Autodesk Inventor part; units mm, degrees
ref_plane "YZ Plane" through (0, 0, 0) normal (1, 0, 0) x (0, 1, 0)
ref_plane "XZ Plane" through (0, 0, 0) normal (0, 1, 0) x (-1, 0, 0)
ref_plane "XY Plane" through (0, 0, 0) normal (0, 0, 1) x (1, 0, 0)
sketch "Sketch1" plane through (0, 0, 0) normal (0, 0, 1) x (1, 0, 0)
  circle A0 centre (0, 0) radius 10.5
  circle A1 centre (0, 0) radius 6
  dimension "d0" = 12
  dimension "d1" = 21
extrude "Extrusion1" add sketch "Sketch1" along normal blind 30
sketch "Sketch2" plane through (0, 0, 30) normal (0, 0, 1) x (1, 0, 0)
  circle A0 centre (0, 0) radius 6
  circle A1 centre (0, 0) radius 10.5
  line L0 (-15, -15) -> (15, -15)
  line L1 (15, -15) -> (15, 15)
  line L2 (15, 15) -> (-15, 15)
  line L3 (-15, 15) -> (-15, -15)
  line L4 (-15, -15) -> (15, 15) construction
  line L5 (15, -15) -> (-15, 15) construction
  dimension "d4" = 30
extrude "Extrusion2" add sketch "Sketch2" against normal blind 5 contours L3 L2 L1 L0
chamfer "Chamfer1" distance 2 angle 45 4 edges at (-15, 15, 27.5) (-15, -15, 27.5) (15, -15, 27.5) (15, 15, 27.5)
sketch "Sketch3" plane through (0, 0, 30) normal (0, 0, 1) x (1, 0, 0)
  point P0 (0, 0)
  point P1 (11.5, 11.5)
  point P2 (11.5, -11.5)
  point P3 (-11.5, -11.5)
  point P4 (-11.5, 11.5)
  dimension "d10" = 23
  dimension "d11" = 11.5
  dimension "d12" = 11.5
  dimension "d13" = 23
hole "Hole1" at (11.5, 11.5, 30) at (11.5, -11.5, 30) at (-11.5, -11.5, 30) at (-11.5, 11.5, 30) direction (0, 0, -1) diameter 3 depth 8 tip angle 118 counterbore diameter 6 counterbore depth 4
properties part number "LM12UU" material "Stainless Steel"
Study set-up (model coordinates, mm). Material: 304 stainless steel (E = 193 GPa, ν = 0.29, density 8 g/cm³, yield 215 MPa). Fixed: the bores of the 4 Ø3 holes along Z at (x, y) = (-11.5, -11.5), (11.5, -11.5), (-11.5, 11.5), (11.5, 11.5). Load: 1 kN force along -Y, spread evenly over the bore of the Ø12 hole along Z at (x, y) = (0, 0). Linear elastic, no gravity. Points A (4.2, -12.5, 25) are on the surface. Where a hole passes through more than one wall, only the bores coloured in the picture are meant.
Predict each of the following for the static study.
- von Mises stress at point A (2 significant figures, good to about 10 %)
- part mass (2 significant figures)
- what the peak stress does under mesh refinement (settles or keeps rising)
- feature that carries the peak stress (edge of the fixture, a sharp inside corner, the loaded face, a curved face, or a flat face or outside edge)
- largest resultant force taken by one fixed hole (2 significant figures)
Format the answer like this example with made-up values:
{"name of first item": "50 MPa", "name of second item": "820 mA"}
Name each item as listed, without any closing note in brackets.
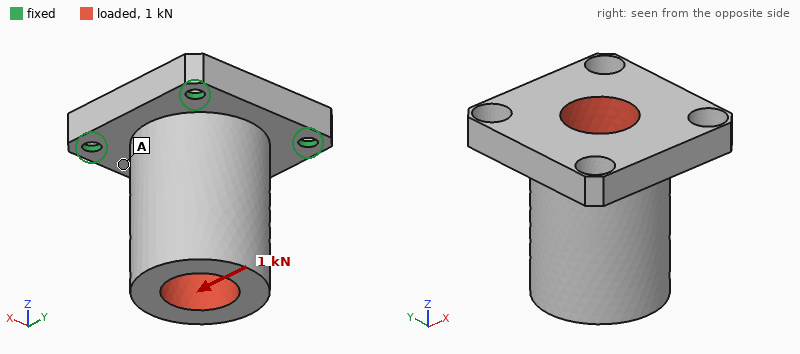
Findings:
{"von Mises stress at point A": "12 MPa", "part mass": "74 g", "what the peak stress does under mesh refinement": "keeps rising", "feature that carries the peak stress": "edge of the fixture", "largest resultant force taken by one fixed hole": "350 N"}
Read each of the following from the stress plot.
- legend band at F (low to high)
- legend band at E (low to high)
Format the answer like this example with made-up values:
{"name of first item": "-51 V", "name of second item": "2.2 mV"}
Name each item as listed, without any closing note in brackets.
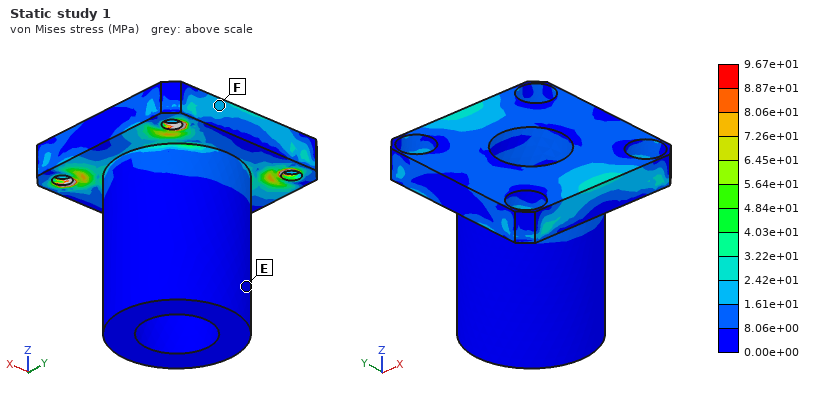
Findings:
{"legend band at F": "1.61e+01 to 2.42e+01 MPa", "legend band at E": "0.00e+00 to 8.06e+00 MPa"}
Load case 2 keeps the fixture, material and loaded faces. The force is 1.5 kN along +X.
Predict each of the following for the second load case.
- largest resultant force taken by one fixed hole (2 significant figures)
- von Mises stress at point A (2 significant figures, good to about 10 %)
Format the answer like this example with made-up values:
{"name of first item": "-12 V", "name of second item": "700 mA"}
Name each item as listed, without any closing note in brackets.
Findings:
{"largest resultant force taken by one fixed hole": "520 N", "von Mises stress at point A": "29 MPa"}
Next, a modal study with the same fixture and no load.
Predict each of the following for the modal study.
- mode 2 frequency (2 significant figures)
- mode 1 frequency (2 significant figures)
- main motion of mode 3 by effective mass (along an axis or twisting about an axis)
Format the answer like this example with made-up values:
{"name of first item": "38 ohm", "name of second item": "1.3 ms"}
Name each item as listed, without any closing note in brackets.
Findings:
{"mode 2 frequency": "7400 Hz", "mode 1 frequency": "7300 Hz", "main motion of mode 3 by effective mass": "along Z"}
